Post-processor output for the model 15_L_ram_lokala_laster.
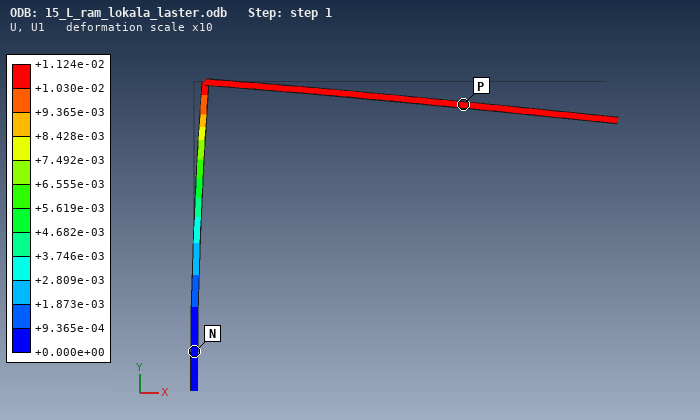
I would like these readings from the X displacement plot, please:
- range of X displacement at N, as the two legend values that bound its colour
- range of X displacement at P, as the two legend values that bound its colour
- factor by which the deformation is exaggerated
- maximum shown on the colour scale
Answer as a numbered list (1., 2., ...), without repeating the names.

1. +0.000e+00 to +9.365e-04
2. +1.030e-02 to +1.124e-02
3. 10
4. +1.124e-02
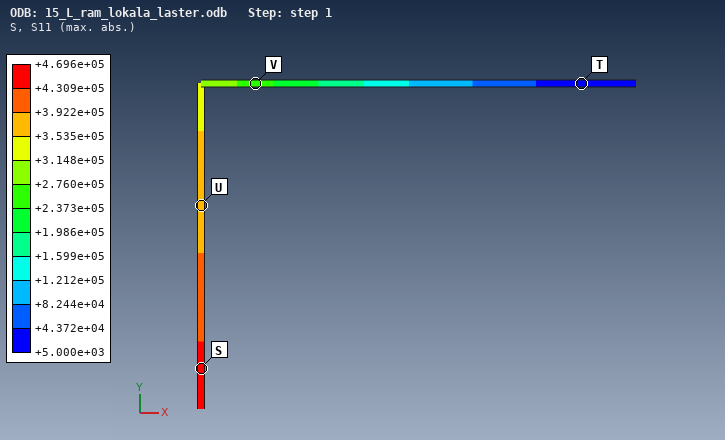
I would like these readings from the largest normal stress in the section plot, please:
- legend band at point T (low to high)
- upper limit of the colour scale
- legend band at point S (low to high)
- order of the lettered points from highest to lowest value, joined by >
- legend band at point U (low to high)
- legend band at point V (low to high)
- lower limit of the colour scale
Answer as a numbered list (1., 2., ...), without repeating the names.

1. +5.000e+03 to +4.372e+04
2. +4.696e+05
3. +4.309e+05 to +4.696e+05
4. S > U > V > T
5. +3.535e+05 to +3.922e+05
6. +2.373e+05 to +2.760e+05
7. +5.000e+03
